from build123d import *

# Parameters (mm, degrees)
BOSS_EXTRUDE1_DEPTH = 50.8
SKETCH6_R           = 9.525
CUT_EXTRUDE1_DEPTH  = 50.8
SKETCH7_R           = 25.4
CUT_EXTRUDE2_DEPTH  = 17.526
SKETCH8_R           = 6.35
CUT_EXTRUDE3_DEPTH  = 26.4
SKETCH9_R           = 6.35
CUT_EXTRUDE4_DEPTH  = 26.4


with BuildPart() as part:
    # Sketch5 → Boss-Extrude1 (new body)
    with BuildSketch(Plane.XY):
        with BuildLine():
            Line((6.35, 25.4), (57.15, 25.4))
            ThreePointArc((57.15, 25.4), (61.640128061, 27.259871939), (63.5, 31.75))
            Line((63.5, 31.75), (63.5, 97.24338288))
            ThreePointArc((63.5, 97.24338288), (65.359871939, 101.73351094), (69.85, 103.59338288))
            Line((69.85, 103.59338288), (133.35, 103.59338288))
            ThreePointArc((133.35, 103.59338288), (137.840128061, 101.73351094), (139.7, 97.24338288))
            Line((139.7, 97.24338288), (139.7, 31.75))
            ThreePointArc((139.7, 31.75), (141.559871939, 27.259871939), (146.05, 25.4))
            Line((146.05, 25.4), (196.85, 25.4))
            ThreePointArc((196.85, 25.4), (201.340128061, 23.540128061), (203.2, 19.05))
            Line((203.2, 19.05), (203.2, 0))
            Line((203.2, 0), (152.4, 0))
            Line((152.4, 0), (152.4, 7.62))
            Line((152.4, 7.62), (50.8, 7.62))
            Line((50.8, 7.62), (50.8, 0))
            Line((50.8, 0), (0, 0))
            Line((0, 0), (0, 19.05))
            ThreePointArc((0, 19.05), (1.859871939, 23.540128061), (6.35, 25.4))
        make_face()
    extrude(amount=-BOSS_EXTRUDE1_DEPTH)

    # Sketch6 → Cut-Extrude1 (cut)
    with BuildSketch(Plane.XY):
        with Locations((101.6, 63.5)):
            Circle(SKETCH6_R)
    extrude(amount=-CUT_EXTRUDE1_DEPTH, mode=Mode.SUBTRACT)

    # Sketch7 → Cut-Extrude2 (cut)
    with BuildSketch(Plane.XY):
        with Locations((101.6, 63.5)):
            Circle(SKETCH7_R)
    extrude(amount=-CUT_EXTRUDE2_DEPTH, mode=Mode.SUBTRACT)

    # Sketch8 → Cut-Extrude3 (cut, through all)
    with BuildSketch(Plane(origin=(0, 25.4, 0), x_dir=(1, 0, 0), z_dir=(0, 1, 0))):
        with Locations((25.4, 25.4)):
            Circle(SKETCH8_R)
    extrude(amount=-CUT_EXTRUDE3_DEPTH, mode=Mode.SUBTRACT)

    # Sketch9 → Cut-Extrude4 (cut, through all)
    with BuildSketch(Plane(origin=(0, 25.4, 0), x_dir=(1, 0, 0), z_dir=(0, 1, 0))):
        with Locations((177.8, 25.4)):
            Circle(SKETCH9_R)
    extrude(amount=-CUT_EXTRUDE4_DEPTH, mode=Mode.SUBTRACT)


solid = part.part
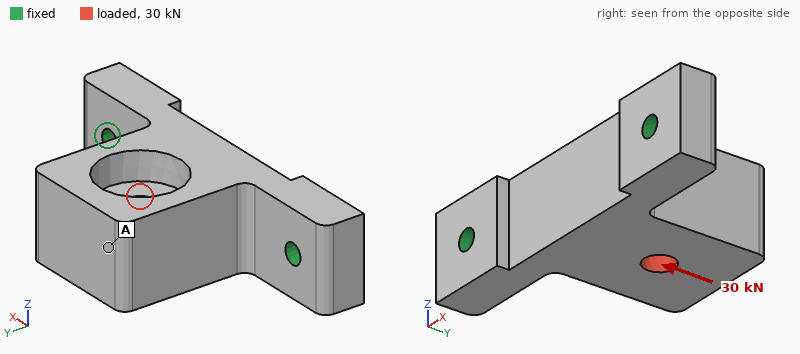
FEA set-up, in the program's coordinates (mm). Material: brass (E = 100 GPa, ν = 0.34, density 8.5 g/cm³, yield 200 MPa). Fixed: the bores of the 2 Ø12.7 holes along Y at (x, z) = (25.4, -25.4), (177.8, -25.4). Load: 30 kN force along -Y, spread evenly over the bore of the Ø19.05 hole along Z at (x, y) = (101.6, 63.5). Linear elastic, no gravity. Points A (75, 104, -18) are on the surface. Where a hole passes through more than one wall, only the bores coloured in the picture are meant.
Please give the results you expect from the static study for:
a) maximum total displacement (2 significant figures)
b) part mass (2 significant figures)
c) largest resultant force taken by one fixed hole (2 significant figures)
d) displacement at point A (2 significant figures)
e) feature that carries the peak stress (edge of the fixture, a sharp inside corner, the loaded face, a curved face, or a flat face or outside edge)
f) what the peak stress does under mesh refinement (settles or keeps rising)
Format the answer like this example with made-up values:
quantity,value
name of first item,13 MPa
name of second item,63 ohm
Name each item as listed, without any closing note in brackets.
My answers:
quantity,value
maximum total displacement,0.12 mm
part mass,4.0 kg
largest resultant force taken by one fixed hole,19 kN
displacement at point A,0.10 mm
feature that carries the peak stress,edge of the fixture
what the peak stress does under mesh refinement,keeps rising
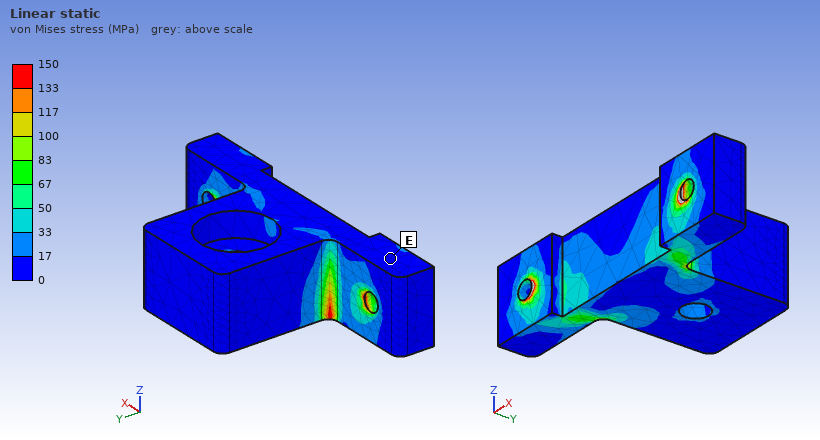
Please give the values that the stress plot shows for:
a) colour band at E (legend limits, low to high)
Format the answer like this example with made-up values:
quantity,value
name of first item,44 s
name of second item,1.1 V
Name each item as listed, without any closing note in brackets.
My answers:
quantity,value
colour band at E,0 to 17 MPa
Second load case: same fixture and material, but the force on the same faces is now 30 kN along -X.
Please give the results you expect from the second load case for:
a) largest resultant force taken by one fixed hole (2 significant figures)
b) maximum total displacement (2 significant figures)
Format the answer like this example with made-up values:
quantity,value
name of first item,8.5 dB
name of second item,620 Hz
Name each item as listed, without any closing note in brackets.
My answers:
quantity,value
largest resultant force taken by one fixed hole,20 kN
maximum total displacement,89 µm
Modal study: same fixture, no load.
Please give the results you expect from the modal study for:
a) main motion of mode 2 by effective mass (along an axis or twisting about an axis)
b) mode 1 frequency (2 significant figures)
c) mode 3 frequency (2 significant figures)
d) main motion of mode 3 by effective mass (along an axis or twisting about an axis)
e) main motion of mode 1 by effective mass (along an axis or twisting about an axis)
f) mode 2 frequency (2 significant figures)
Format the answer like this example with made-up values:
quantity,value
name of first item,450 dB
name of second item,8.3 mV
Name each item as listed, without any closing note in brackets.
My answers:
quantity,value
main motion of mode 2 by effective mass,along X
mode 1 frequency,870 Hz
mode 3 frequency,2400 Hz
main motion of mode 3 by effective mass,along Y
main motion of mode 1 by effective mass,along Z
mode 2 frequency,2200 Hz
